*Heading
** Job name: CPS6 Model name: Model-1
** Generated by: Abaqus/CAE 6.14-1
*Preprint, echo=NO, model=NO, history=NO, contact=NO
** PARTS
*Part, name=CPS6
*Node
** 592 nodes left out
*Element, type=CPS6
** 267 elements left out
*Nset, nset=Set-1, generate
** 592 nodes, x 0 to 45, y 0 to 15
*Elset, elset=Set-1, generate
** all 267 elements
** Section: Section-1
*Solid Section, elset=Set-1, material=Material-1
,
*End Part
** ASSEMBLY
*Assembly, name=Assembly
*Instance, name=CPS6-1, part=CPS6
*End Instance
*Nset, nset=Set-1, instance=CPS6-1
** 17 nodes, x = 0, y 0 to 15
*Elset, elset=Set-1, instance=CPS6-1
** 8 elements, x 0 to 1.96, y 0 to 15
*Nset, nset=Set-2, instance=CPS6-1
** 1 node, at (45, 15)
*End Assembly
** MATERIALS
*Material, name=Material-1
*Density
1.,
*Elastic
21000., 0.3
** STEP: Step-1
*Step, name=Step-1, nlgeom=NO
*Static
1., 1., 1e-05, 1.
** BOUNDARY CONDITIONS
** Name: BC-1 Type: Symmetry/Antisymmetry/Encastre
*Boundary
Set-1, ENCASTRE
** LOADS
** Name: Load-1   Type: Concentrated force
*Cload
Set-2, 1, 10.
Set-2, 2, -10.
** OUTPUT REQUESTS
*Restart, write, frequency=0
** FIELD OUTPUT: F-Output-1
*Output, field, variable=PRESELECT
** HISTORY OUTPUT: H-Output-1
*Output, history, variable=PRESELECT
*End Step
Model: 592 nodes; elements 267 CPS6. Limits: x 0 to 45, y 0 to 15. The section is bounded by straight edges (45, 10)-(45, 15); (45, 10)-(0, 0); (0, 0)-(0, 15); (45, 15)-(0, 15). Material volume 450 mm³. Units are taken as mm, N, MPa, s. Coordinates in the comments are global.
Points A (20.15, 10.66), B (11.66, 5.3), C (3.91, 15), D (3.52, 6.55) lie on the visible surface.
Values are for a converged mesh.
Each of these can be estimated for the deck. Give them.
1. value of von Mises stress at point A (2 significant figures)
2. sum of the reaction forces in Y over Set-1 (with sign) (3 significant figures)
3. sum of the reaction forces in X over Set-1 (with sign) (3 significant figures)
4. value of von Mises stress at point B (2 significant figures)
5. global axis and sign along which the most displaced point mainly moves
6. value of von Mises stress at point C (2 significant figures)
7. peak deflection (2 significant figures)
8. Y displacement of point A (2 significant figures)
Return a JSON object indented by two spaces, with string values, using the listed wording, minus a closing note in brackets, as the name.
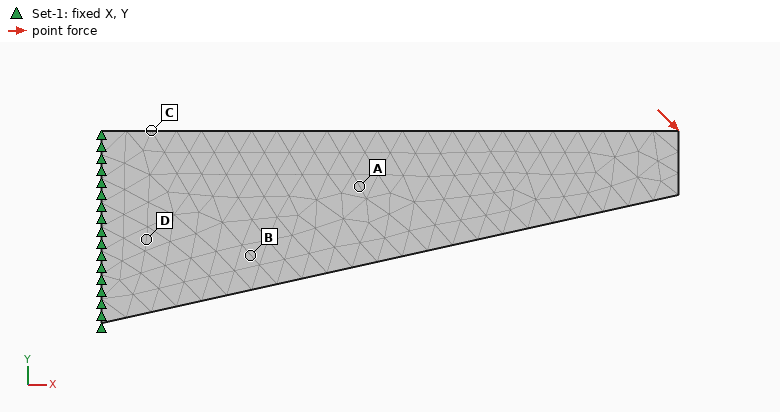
{
  "value of von Mises stress at point A": "3.8 MPa",
  "sum of the reaction forces in Y over Set-1 (with sign)": "10.0 N",
  "sum of the reaction forces in X over Set-1 (with sign)": "-10.0 N",
  "value of von Mises stress at point B": "8.3 MPa",
  "global axis and sign along which the most displaced point mainly moves": "-Y",
  "value of von Mises stress at point C": "15 MPa",
  "peak deflection": "0.15 mm",
  "Y displacement of point A": "-0.023 mm"
}
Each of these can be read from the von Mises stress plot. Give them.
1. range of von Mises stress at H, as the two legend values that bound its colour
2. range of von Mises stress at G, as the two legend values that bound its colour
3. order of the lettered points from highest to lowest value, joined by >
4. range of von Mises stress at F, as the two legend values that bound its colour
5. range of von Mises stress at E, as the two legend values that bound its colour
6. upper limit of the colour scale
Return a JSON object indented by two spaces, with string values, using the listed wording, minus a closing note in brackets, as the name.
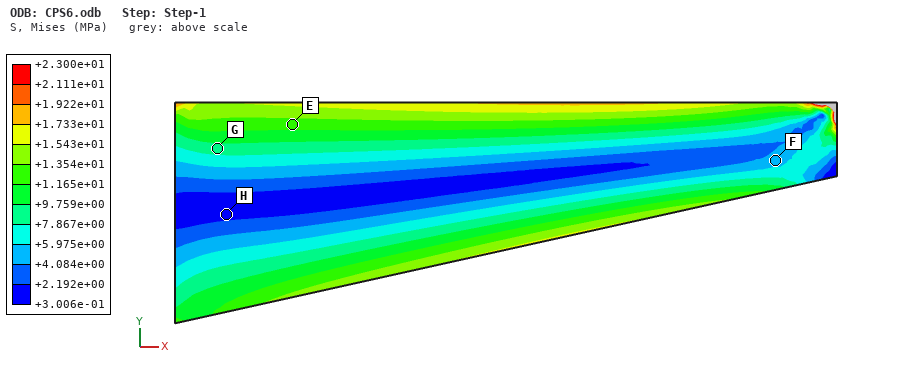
{
  "range of von Mises stress at H, as the two legend values that bound its colour": "+3.006e-01 to +2.192e+00 MPa",
  "range of von Mises stress at G, as the two legend values that bound its colour": "+7.867e+00 to +9.759e+00 MPa",
  "order of the lettered points from highest to lowest value, joined by >": "E > G > F > H",
  "range of von Mises stress at F, as the two legend values that bound its colour": "+4.084e+00 to +5.975e+00 MPa",
  "range of von Mises stress at E, as the two legend values that bound its colour": "+1.165e+01 to +1.354e+01 MPa",
  "upper limit of the colour scale": "+2.300e+01 MPa"
}
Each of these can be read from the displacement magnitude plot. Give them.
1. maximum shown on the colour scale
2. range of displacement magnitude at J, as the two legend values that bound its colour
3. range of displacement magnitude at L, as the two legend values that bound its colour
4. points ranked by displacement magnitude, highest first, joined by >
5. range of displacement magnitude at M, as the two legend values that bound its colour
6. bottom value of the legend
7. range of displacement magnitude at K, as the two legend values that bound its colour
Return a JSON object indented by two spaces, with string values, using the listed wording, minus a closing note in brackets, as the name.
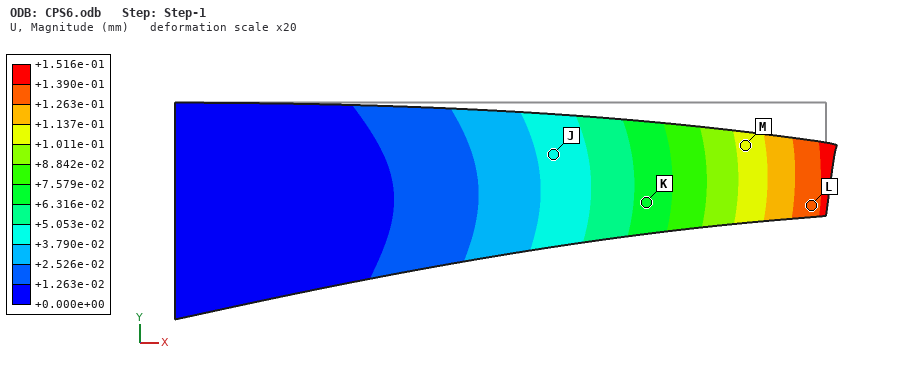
{
  "maximum shown on the colour scale": "+1.516e-01 mm",
  "range of displacement magnitude at J, as the two legend values that bound its colour": "+3.790e-02 to +5.053e-02 mm",
  "range of displacement magnitude at L, as the two legend values that bound its colour": "+1.263e-01 to +1.390e-01 mm",
  "points ranked by displacement magnitude, highest first, joined by >": "L > M > K > J",
  "range of displacement magnitude at M, as the two legend values that bound its colour": "+1.011e-01 to +1.137e-01 mm",
  "bottom value of the legend": "+0.000e+00 mm",
  "range of displacement magnitude at K, as the two legend values that bound its colour": "+6.316e-02 to +7.579e-02 mm"
}
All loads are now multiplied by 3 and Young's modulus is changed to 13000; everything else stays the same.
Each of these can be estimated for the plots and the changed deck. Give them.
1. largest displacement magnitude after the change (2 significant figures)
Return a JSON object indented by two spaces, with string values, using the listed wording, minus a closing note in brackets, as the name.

{
  "largest displacement magnitude after the change": "0.73 mm"
}
